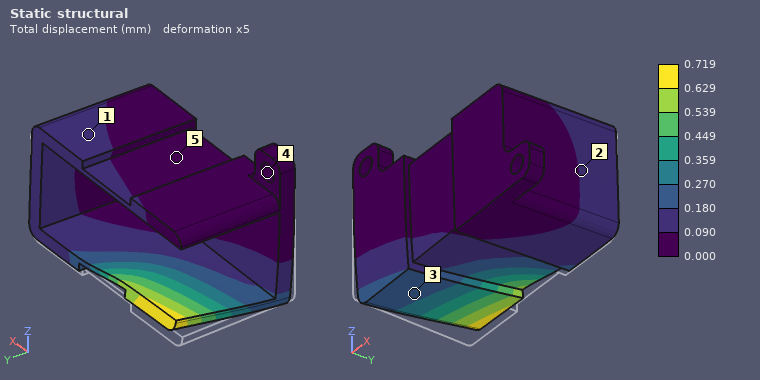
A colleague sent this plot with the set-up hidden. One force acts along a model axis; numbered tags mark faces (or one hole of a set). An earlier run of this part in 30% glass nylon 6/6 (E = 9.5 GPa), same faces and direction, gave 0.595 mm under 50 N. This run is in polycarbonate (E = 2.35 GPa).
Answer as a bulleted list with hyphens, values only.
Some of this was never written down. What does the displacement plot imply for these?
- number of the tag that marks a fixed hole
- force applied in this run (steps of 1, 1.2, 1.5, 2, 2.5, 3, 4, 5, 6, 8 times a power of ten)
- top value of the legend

- 4
- 15 N
- 0.719 mm
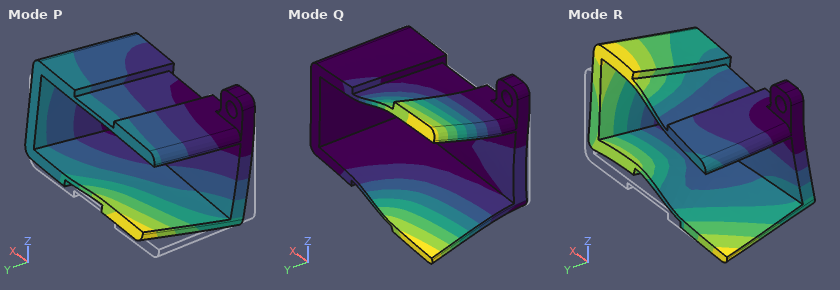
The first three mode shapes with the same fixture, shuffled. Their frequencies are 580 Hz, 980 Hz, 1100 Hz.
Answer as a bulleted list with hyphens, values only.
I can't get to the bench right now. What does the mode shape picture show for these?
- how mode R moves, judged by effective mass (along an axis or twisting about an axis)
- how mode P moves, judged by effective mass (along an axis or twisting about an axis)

- along Y
- along Z
